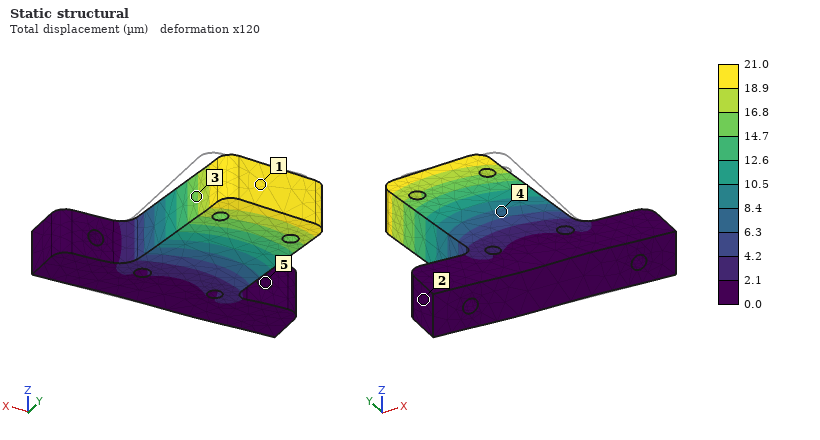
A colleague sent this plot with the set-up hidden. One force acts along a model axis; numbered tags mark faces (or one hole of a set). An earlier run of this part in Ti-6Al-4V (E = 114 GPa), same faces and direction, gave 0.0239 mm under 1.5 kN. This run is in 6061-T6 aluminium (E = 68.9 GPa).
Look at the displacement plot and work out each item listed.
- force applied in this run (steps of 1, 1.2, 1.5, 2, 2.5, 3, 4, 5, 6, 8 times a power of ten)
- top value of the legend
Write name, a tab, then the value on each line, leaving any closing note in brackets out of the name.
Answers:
force applied in this run	800 N
top value of the legend	21.0 µm
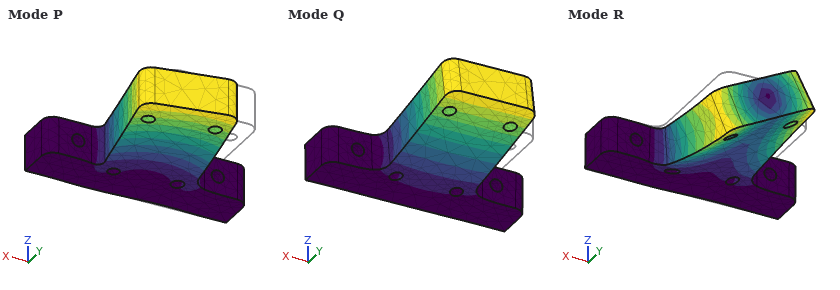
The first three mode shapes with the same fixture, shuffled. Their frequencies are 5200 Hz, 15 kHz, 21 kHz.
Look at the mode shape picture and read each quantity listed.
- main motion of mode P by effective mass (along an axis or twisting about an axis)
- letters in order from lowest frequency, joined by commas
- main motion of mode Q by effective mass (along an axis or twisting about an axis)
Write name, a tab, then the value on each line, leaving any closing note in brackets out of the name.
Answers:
main motion of mode P by effective mass	along X
letters in order from lowest frequency, joined by commas	Q, P, R
main motion of mode Q by effective mass	along Z
